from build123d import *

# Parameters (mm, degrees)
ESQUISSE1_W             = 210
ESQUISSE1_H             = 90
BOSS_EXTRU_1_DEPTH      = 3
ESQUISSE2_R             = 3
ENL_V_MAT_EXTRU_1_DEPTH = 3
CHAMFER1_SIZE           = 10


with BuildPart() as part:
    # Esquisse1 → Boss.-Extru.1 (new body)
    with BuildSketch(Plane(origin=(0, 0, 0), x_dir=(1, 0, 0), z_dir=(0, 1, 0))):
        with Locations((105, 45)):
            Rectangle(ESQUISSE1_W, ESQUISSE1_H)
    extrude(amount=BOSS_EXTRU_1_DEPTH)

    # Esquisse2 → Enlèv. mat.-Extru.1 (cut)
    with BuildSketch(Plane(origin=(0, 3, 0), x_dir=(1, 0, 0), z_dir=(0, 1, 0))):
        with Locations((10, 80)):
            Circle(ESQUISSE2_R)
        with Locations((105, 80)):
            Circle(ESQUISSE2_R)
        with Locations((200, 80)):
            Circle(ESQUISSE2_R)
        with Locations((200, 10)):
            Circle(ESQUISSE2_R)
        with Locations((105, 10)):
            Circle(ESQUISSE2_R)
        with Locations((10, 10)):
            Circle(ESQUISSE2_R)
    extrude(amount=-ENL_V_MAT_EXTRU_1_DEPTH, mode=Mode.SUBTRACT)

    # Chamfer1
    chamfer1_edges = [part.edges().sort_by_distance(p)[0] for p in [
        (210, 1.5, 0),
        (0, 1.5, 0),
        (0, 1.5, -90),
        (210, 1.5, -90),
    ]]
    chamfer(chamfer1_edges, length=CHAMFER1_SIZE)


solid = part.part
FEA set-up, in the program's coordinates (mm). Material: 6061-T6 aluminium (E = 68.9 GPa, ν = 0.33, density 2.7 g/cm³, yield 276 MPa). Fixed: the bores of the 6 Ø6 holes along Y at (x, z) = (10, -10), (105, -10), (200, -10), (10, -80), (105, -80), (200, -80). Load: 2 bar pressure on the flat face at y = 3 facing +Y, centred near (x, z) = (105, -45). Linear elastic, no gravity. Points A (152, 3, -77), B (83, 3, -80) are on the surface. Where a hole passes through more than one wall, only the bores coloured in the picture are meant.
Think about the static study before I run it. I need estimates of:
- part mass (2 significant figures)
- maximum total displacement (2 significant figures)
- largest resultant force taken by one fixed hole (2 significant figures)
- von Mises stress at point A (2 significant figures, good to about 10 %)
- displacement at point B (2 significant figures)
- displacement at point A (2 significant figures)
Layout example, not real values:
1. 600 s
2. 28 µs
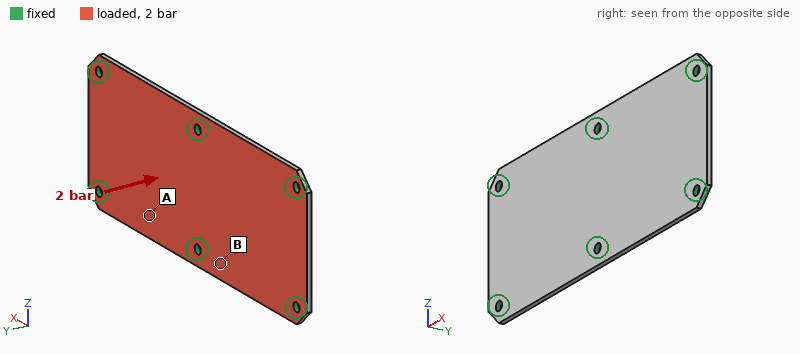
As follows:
1. 150 g
2. 0.36 mm
3. 880 N
4. 50 MPa
5. 0.14 mm
6. 0.30 mm
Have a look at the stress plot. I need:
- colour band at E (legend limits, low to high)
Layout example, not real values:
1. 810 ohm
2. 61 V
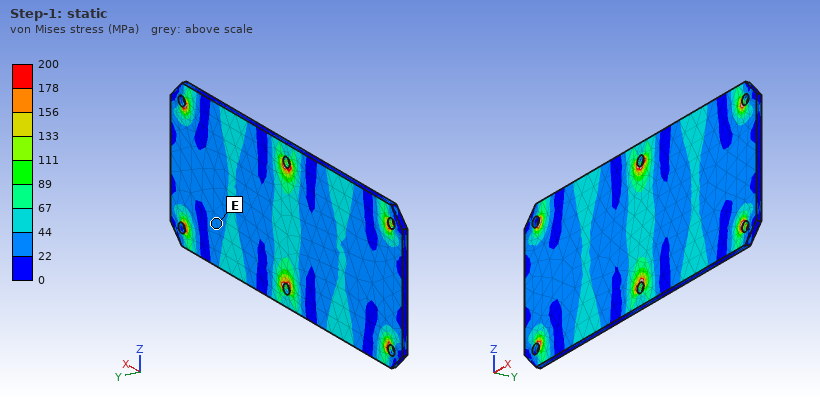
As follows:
1. 22 to 44 MPa
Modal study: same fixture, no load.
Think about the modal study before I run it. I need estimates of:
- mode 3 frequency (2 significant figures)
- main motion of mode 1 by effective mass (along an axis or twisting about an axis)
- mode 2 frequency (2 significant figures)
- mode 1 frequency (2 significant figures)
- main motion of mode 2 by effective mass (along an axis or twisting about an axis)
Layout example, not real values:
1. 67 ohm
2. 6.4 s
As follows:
1. 2200 Hz
2. twisting about Z
3. 1600 Hz
4. 1500 Hz
5. along Y
